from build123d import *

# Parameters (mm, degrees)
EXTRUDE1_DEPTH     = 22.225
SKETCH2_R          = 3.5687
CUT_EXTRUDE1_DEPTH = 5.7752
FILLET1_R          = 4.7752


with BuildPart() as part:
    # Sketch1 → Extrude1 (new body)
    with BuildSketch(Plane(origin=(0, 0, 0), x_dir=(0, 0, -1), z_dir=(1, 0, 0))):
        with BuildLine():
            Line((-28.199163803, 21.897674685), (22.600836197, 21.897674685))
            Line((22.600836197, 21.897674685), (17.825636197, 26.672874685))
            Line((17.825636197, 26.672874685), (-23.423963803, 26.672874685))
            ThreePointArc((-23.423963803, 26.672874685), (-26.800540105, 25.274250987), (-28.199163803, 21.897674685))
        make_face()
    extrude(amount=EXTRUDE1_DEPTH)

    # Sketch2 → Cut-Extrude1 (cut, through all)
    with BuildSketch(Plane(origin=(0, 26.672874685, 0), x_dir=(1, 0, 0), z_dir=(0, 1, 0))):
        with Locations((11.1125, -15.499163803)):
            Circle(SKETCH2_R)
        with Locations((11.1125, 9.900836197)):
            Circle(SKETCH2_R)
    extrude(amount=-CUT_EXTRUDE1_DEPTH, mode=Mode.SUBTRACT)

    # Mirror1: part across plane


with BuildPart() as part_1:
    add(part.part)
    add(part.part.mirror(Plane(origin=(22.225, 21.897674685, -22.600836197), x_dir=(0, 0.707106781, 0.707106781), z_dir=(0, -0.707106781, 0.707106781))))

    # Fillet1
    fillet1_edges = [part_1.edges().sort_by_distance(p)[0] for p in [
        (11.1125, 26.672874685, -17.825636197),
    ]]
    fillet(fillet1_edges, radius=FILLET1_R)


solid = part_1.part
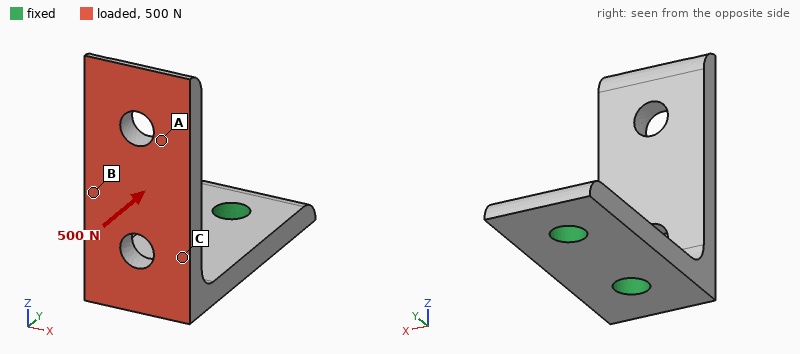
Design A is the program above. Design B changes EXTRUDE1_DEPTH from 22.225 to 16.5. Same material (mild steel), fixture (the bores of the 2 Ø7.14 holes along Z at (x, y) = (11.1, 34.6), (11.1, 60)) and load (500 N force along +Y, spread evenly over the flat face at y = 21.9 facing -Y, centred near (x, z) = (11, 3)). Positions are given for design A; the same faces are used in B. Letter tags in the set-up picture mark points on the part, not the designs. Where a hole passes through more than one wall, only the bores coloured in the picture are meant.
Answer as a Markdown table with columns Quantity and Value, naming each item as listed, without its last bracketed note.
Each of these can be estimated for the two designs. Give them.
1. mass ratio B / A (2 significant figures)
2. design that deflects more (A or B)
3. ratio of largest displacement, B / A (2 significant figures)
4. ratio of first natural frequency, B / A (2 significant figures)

| Quantity | Value |
|---|---|
| mass ratio B / A | 0.72 |
| design that deflects more | B |
| ratio of largest displacement, B / A | 1.4 |
| ratio of first natural frequency, B / A | 0.98 |
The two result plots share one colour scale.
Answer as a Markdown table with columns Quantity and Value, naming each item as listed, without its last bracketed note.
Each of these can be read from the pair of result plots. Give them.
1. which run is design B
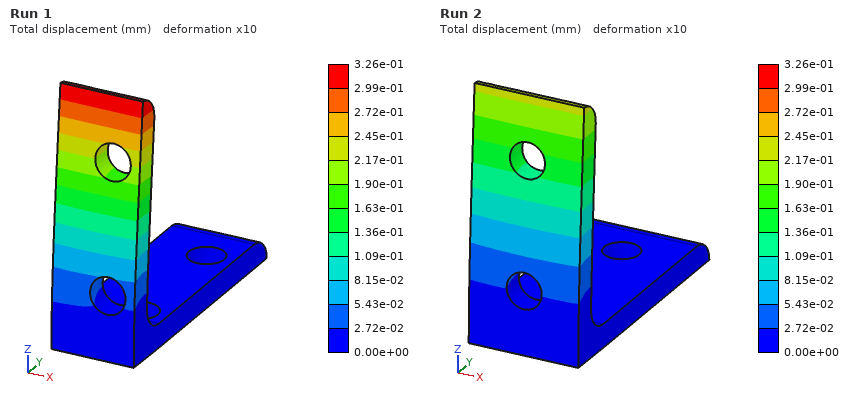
| Quantity | Value |
|---|---|
| which run is design B | Run 1 |
